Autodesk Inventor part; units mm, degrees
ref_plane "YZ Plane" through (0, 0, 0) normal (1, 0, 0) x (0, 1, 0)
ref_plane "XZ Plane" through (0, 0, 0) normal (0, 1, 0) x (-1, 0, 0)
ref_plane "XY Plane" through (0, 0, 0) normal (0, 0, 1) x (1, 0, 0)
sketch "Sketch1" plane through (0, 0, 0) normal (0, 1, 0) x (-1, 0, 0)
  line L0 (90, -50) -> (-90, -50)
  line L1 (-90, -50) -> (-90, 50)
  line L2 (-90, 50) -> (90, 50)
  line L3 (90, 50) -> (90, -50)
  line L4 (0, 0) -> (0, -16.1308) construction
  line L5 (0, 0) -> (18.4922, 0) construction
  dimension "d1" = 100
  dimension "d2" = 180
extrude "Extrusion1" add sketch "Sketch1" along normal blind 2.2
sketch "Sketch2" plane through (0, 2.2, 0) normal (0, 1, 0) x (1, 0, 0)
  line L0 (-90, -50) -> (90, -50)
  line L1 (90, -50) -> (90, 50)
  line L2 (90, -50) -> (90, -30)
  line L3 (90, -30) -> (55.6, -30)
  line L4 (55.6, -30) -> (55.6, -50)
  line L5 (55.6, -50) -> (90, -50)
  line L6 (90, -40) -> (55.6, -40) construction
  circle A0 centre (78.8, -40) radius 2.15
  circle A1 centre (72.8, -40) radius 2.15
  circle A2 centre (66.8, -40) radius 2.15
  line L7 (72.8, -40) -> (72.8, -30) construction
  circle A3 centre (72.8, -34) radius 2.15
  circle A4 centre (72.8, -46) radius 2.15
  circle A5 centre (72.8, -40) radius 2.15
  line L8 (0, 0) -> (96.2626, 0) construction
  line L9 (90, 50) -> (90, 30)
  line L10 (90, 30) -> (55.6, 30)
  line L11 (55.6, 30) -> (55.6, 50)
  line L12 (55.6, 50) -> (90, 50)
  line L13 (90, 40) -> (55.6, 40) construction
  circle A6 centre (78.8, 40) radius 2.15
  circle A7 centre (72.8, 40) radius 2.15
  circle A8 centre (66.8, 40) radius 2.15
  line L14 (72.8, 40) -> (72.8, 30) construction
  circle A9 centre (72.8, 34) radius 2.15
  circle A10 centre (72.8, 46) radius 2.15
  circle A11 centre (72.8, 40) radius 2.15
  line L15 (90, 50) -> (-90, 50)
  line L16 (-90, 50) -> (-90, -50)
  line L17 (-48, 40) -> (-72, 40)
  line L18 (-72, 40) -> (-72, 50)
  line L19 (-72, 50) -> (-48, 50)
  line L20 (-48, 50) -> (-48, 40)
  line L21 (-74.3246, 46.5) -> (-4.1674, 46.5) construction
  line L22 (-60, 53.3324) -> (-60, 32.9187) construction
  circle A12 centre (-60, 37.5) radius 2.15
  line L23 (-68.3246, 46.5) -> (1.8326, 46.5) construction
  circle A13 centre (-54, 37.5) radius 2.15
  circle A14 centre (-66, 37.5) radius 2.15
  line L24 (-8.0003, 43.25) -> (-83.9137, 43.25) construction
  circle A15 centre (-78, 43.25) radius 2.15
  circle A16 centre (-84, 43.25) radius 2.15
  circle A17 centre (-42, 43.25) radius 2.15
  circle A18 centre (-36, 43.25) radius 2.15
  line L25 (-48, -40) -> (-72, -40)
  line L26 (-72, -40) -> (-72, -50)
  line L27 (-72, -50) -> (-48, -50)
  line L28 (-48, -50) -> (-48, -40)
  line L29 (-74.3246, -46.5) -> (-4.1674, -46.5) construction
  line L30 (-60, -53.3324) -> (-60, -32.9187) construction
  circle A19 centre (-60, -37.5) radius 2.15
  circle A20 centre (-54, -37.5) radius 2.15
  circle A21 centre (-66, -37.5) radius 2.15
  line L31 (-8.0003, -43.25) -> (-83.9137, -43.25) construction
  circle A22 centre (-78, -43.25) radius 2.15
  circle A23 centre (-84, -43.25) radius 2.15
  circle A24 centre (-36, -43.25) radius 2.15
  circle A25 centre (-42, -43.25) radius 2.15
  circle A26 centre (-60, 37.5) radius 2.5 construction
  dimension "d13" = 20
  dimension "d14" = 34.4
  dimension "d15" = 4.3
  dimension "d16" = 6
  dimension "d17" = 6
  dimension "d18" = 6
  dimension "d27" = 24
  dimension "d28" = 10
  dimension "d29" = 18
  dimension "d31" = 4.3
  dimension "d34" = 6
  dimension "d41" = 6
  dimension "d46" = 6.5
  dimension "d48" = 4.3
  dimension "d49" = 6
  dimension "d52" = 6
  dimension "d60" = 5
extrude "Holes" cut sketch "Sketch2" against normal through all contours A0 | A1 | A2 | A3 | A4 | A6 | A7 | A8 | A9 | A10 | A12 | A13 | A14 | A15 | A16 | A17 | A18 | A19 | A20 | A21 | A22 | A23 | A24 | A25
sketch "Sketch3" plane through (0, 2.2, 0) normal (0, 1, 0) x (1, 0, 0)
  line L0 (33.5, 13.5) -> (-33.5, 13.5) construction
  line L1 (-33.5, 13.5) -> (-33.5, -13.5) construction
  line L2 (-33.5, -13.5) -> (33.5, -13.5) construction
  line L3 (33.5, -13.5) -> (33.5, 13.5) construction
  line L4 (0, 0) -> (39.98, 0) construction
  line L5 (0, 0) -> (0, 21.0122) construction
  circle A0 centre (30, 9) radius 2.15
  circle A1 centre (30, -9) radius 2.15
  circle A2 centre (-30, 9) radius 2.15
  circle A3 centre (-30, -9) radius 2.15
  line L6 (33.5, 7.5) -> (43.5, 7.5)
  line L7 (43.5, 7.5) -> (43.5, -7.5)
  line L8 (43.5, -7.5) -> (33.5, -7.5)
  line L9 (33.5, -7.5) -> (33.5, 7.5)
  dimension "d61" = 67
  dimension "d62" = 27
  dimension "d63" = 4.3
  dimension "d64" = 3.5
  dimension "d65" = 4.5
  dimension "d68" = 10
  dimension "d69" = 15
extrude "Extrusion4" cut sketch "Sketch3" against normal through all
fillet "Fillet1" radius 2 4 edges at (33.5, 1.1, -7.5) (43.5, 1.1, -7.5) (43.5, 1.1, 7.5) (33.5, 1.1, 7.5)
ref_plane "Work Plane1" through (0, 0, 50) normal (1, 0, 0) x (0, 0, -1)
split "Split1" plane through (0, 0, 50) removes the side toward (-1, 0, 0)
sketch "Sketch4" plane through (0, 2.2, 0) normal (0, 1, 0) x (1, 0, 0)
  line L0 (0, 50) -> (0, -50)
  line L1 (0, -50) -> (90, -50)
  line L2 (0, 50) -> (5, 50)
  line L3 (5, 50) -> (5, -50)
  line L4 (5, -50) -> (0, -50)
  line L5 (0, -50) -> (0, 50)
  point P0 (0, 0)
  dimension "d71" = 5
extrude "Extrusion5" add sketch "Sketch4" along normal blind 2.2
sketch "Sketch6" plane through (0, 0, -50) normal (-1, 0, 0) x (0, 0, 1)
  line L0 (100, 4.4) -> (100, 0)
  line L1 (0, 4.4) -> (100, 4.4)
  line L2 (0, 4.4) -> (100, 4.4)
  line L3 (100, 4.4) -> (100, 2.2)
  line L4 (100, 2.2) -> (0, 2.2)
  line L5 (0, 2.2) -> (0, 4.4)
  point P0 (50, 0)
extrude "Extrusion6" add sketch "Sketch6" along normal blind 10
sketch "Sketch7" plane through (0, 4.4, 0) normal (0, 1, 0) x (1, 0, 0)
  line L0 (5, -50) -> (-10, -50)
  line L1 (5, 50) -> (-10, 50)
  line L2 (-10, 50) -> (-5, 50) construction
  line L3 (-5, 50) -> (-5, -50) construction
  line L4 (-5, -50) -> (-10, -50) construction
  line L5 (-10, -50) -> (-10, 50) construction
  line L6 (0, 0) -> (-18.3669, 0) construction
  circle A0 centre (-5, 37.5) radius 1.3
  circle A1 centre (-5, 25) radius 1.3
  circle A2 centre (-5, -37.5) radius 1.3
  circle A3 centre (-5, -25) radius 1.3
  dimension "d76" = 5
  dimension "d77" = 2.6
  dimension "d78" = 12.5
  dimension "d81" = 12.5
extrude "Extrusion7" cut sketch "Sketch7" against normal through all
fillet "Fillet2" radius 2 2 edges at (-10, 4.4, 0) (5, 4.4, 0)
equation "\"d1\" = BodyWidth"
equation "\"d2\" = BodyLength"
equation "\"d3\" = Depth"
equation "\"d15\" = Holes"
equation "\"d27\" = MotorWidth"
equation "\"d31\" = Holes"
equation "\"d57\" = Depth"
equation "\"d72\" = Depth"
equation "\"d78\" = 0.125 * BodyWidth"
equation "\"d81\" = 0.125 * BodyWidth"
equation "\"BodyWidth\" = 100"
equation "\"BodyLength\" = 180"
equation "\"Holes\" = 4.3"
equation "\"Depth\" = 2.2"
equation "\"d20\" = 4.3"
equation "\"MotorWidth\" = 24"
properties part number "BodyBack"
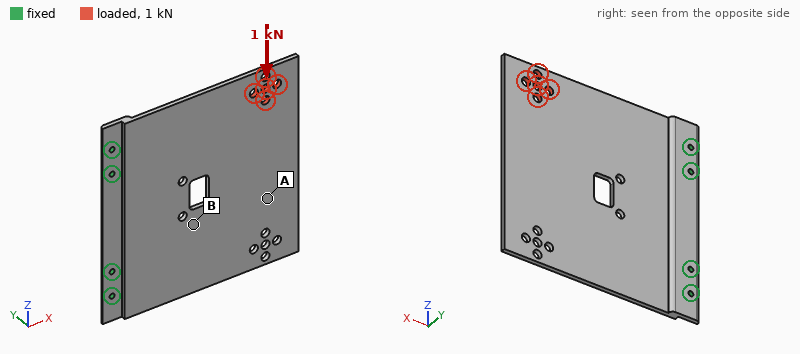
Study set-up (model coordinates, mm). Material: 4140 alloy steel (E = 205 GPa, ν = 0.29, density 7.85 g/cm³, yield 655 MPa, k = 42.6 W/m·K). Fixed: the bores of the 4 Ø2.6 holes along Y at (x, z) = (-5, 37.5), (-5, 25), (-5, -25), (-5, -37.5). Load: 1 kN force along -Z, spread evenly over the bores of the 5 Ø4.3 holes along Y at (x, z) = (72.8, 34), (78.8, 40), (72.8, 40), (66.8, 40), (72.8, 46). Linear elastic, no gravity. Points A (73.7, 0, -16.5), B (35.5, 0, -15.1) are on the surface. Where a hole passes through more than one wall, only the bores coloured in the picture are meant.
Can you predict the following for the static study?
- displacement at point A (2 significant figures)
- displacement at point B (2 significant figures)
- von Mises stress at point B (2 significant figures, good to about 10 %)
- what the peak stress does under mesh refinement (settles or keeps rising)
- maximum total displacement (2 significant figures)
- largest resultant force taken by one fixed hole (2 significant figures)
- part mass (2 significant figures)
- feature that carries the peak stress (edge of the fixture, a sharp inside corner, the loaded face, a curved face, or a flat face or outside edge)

29 µm
19 µm
12 MPa
keeps rising
73 µm
850 N
170 g
edge of the fixture
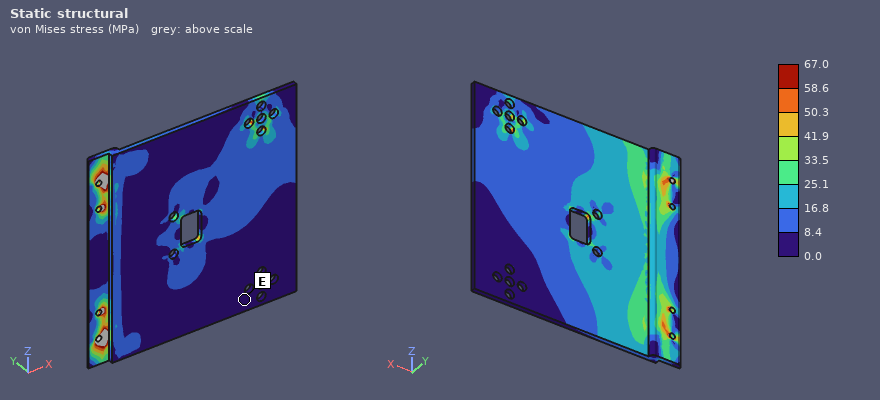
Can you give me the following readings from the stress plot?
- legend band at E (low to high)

0.0 to 8.4 MPa
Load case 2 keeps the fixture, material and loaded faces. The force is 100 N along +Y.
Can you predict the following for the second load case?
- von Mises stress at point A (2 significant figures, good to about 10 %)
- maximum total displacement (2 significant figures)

27 MPa
1.6 mm
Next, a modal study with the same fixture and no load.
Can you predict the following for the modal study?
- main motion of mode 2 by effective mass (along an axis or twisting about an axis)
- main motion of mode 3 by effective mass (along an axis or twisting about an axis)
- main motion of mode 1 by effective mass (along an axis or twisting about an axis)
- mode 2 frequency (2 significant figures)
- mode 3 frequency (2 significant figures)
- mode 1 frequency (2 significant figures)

twisting about X
along Y
along Y
500 Hz
1200 Hz
200 Hz
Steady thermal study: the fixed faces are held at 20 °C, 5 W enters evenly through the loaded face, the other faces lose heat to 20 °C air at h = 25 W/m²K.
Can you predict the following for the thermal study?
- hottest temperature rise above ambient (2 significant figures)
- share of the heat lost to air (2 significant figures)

43 K
81 %
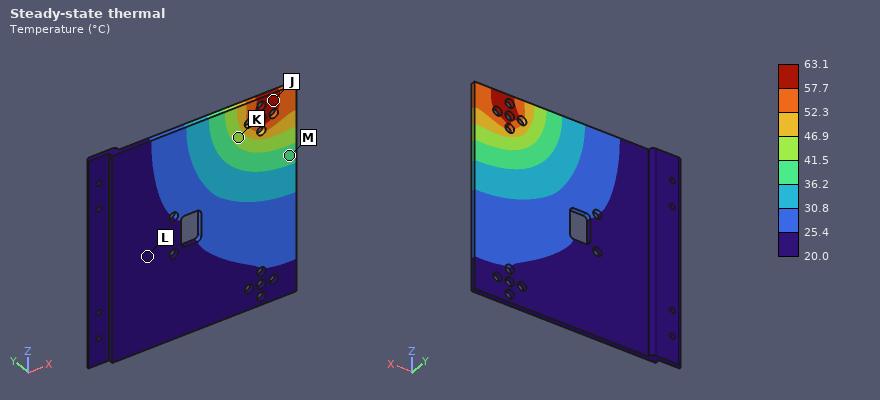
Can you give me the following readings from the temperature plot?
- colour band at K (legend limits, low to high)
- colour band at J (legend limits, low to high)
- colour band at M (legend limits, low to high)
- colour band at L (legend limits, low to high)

41.5 to 46.9 °C
57.7 to 63.1 °C
36.2 to 41.5 °C
20.0 to 25.4 °C
